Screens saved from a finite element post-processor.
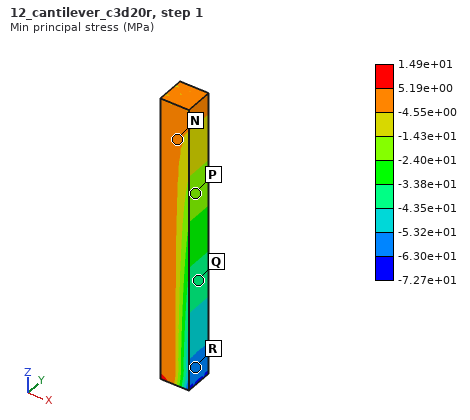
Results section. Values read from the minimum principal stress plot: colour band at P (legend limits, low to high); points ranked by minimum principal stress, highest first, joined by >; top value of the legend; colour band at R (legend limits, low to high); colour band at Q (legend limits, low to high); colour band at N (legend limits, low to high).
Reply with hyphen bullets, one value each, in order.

- -2.40e+01 to -1.43e+01 MPa
- N > P > Q > R
- 1.49e+01 MPa
- -6.30e+01 to -5.32e+01 MPa
- -4.35e+01 to -3.38e+01 MPa
- -4.55e+00 to 5.19e+00 MPa
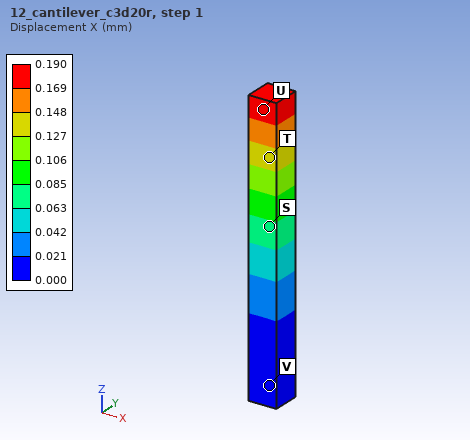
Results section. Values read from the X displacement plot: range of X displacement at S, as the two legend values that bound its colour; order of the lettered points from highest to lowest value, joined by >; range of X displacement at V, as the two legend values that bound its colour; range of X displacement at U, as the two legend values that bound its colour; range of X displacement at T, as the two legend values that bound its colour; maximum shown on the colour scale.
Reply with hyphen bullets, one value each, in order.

- 0.063 to 0.085 mm
- U > T > S > V
- 0.000 to 0.021 mm
- 0.169 to 0.190 mm
- 0.127 to 0.148 mm
- 0.190 mm
